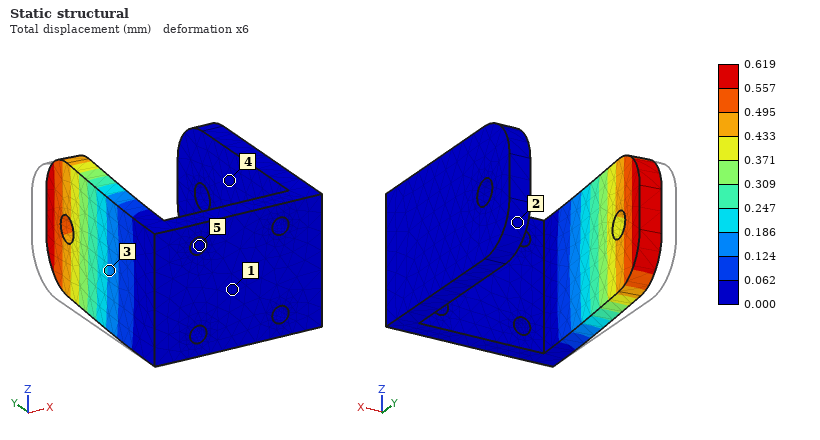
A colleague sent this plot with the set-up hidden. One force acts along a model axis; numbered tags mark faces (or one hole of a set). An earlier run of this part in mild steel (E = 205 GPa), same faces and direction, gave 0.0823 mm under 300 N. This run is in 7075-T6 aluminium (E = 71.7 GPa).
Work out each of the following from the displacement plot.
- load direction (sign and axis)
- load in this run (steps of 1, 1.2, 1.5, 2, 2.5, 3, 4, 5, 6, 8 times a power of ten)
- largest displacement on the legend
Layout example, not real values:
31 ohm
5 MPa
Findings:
+X
800 N
0.619 mm
